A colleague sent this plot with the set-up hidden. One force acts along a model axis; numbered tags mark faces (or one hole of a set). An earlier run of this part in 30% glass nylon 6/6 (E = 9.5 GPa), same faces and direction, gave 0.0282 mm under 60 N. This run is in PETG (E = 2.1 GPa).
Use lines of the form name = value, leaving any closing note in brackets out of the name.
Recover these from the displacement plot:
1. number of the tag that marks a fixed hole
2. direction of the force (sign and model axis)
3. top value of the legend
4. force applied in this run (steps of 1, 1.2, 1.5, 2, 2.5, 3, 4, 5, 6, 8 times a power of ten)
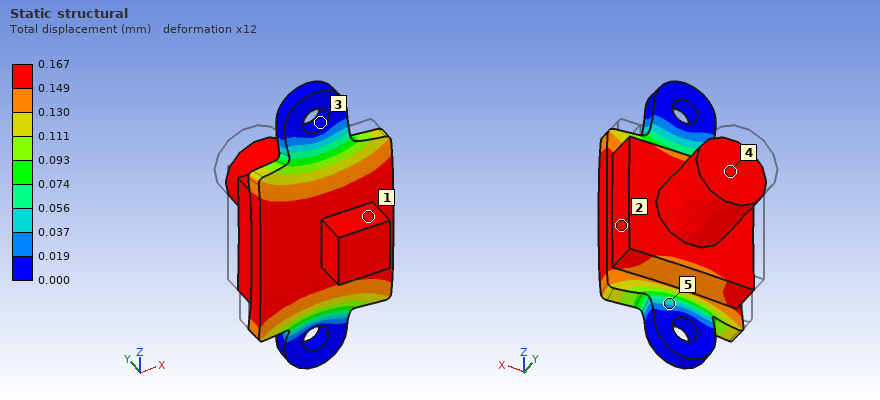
number of the tag that marks a fixed hole = 3
direction of the force = -Y
top value of the legend = 0.167 mm
force applied in this run = 80 N
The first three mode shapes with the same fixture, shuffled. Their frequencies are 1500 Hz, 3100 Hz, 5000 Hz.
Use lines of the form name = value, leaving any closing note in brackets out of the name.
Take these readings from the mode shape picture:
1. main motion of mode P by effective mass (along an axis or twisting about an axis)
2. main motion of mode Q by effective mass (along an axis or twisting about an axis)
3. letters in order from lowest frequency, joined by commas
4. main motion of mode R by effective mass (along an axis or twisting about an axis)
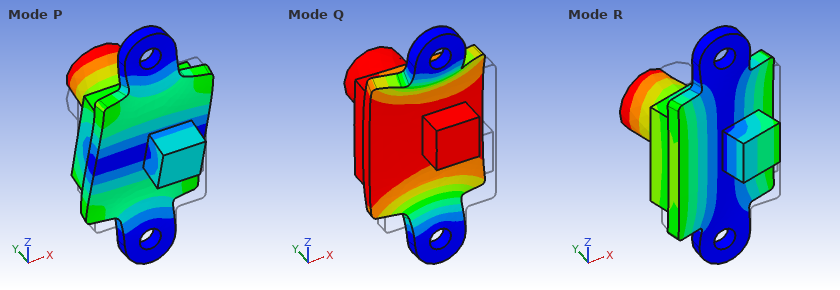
main motion of mode P by effective mass = along Z
main motion of mode Q by effective mass = along Y
letters in order from lowest frequency, joined by commas = R, Q, P
main motion of mode R by effective mass = along X
